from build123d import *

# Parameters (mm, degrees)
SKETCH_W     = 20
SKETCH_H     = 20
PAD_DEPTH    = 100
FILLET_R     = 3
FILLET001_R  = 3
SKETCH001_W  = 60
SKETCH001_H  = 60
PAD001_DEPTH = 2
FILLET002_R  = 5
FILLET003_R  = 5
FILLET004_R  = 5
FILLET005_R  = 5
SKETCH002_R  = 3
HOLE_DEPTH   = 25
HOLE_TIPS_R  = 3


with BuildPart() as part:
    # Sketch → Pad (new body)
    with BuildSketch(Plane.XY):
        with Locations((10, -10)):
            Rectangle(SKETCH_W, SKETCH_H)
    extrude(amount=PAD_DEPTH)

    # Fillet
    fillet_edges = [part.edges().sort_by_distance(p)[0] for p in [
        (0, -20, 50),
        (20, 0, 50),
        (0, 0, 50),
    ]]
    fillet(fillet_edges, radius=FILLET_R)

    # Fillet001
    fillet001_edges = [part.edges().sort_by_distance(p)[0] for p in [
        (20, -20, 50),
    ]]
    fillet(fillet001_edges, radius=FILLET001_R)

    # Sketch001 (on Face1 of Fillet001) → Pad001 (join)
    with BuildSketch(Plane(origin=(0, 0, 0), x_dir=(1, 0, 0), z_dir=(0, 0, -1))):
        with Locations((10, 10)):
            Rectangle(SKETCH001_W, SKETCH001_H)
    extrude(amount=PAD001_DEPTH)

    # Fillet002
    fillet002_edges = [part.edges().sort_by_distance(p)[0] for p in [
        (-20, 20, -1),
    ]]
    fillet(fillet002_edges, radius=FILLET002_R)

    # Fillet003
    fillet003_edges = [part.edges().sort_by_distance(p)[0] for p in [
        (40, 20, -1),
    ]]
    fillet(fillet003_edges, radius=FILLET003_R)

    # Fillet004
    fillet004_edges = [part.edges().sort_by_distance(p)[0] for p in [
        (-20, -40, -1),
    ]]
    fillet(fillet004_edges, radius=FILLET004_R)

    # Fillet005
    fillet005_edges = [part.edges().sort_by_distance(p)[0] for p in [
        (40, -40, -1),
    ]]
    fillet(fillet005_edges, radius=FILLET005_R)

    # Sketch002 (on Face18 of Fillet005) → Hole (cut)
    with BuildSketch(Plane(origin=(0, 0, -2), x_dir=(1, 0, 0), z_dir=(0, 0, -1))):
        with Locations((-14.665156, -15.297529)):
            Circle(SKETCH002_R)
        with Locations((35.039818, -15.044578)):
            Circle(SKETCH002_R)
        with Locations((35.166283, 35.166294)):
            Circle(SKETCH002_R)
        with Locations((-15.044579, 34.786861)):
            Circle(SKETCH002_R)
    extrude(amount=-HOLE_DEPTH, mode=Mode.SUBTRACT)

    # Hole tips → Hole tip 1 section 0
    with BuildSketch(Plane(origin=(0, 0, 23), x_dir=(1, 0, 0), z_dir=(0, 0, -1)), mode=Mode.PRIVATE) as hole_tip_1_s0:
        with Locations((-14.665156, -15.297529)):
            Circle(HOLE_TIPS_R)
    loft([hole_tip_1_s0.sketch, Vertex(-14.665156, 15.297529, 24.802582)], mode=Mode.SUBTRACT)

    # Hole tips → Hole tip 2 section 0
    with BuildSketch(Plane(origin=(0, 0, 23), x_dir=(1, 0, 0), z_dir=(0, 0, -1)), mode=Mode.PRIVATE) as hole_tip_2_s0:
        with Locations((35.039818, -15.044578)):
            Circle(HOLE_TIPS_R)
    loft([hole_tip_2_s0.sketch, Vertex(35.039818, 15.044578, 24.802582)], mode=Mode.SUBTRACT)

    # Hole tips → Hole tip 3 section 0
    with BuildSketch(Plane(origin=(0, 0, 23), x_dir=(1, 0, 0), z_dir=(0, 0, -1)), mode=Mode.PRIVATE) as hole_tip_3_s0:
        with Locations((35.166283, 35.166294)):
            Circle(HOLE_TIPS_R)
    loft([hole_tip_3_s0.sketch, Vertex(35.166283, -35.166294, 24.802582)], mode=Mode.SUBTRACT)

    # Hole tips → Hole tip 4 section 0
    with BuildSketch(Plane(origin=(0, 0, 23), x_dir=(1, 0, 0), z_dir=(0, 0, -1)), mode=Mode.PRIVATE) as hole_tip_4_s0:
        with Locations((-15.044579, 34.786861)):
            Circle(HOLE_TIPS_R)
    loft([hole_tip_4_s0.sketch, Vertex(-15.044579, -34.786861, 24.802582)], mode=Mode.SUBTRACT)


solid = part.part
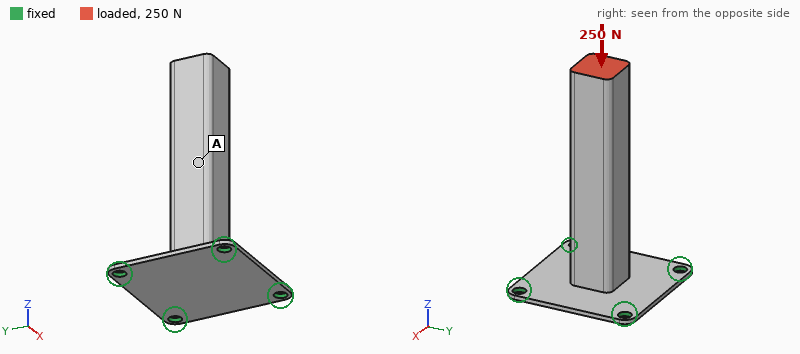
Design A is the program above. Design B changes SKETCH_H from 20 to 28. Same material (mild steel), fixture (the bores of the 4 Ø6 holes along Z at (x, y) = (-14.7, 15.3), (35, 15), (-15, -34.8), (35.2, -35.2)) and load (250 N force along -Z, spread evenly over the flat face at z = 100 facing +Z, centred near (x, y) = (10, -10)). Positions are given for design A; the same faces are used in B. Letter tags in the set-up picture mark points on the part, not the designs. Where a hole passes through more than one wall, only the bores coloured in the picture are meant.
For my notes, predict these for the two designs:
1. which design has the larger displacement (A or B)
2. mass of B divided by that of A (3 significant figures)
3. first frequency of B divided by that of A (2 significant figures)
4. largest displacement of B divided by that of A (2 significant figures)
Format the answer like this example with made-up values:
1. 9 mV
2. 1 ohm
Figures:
1. A
2. 1.35
3. 0.98
4. 0.74
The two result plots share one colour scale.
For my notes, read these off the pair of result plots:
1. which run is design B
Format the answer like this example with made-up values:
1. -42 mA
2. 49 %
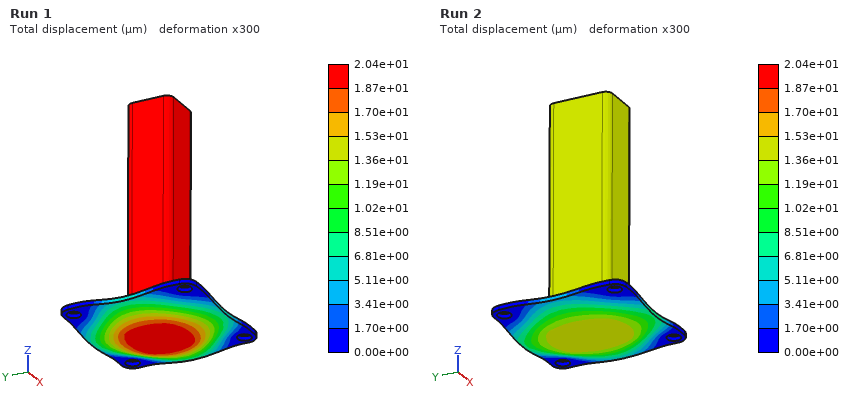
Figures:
1. Run 2
